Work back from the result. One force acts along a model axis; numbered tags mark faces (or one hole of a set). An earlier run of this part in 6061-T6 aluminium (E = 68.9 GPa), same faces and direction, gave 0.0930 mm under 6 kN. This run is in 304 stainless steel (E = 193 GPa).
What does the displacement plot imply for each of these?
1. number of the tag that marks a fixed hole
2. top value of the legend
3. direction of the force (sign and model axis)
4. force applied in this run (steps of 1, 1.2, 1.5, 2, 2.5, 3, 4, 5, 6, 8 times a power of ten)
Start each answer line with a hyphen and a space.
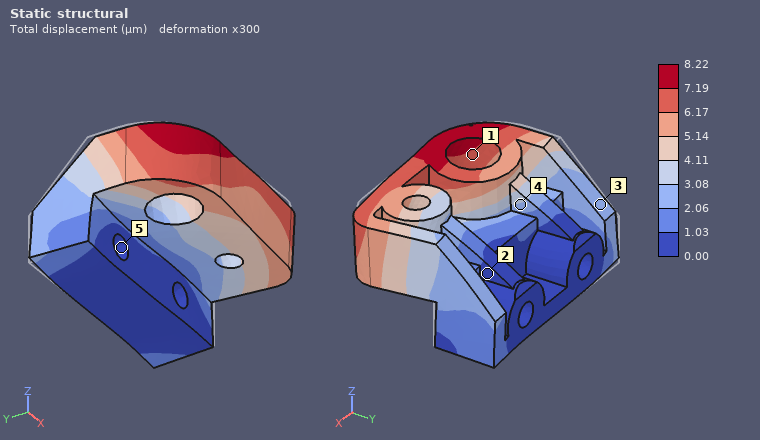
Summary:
- 5
- 8.22 µm
- +X
- 1.5 kN
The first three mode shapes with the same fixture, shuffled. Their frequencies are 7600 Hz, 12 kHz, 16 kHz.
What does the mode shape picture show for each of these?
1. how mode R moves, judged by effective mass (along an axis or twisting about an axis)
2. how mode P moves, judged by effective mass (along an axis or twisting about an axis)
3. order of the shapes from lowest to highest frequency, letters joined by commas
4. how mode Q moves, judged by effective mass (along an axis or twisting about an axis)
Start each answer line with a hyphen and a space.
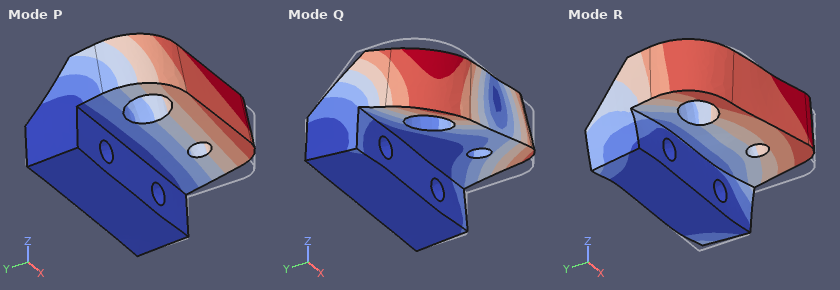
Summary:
- along X
- along Z
- P, Q, R
- twisting about Y
